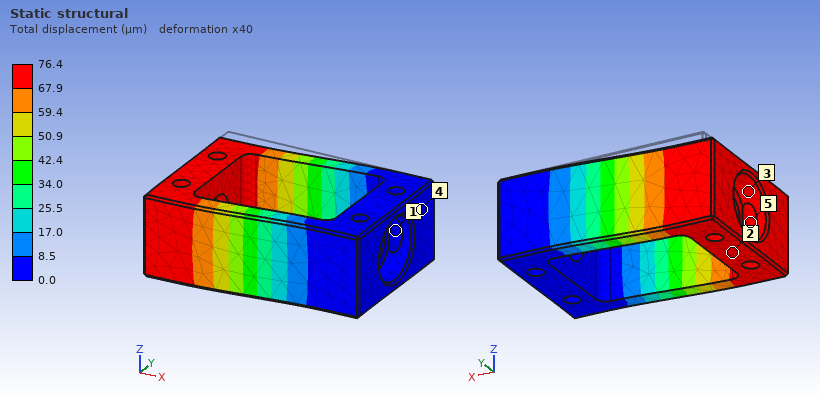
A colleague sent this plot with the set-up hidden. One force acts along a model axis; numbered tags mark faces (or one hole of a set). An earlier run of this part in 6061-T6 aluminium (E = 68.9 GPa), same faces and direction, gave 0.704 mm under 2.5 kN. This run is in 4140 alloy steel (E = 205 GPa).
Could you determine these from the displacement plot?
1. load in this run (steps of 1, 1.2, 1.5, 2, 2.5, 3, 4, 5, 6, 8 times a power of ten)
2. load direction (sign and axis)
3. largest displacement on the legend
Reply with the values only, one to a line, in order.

800 N
-Y
76.4 µm
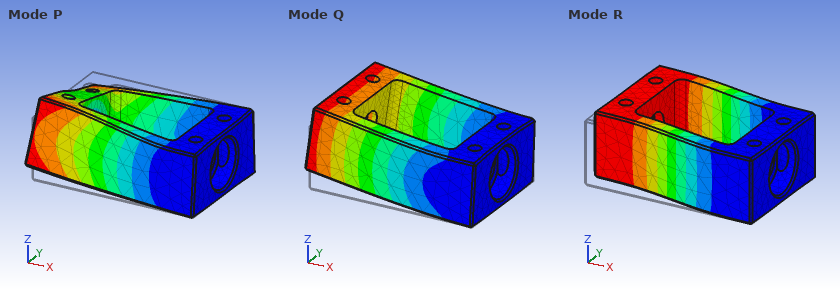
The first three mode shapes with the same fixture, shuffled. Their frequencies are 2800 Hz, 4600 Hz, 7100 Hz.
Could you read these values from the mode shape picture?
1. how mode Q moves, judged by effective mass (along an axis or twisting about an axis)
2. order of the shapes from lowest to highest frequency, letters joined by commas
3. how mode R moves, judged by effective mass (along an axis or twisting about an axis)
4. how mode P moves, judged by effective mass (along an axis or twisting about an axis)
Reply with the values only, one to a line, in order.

along Z
R, Q, P
along Y
twisting about X
